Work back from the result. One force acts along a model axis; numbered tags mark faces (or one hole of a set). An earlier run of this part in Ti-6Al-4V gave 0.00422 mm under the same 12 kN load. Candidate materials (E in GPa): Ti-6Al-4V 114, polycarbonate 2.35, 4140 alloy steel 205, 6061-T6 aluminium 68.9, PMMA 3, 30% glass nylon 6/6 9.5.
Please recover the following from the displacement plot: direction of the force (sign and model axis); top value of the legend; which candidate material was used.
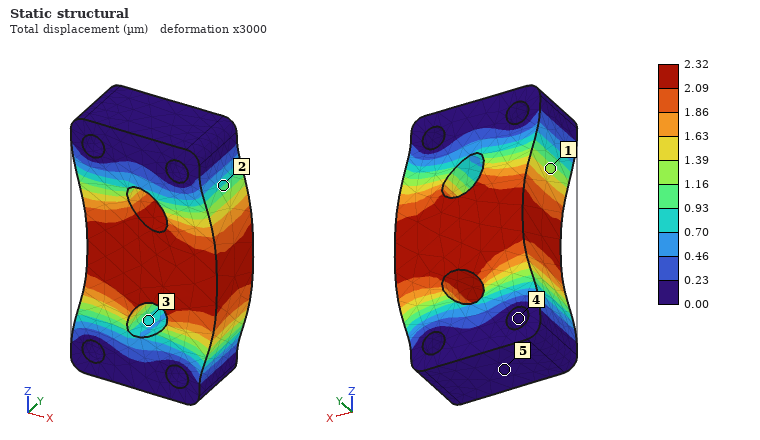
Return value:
+X
2.32 µm
4140 alloy steel
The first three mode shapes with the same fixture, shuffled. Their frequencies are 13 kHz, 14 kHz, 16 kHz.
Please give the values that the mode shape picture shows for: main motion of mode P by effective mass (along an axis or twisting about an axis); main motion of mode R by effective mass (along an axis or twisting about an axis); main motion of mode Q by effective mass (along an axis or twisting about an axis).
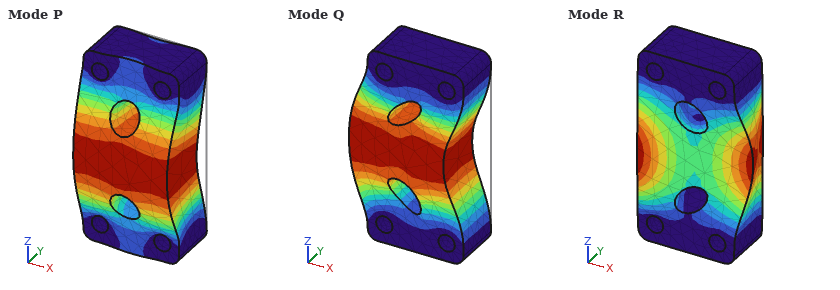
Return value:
along Y
twisting about Z
along X
